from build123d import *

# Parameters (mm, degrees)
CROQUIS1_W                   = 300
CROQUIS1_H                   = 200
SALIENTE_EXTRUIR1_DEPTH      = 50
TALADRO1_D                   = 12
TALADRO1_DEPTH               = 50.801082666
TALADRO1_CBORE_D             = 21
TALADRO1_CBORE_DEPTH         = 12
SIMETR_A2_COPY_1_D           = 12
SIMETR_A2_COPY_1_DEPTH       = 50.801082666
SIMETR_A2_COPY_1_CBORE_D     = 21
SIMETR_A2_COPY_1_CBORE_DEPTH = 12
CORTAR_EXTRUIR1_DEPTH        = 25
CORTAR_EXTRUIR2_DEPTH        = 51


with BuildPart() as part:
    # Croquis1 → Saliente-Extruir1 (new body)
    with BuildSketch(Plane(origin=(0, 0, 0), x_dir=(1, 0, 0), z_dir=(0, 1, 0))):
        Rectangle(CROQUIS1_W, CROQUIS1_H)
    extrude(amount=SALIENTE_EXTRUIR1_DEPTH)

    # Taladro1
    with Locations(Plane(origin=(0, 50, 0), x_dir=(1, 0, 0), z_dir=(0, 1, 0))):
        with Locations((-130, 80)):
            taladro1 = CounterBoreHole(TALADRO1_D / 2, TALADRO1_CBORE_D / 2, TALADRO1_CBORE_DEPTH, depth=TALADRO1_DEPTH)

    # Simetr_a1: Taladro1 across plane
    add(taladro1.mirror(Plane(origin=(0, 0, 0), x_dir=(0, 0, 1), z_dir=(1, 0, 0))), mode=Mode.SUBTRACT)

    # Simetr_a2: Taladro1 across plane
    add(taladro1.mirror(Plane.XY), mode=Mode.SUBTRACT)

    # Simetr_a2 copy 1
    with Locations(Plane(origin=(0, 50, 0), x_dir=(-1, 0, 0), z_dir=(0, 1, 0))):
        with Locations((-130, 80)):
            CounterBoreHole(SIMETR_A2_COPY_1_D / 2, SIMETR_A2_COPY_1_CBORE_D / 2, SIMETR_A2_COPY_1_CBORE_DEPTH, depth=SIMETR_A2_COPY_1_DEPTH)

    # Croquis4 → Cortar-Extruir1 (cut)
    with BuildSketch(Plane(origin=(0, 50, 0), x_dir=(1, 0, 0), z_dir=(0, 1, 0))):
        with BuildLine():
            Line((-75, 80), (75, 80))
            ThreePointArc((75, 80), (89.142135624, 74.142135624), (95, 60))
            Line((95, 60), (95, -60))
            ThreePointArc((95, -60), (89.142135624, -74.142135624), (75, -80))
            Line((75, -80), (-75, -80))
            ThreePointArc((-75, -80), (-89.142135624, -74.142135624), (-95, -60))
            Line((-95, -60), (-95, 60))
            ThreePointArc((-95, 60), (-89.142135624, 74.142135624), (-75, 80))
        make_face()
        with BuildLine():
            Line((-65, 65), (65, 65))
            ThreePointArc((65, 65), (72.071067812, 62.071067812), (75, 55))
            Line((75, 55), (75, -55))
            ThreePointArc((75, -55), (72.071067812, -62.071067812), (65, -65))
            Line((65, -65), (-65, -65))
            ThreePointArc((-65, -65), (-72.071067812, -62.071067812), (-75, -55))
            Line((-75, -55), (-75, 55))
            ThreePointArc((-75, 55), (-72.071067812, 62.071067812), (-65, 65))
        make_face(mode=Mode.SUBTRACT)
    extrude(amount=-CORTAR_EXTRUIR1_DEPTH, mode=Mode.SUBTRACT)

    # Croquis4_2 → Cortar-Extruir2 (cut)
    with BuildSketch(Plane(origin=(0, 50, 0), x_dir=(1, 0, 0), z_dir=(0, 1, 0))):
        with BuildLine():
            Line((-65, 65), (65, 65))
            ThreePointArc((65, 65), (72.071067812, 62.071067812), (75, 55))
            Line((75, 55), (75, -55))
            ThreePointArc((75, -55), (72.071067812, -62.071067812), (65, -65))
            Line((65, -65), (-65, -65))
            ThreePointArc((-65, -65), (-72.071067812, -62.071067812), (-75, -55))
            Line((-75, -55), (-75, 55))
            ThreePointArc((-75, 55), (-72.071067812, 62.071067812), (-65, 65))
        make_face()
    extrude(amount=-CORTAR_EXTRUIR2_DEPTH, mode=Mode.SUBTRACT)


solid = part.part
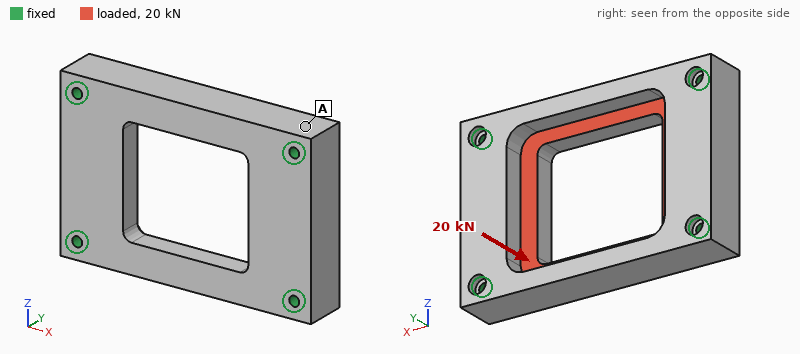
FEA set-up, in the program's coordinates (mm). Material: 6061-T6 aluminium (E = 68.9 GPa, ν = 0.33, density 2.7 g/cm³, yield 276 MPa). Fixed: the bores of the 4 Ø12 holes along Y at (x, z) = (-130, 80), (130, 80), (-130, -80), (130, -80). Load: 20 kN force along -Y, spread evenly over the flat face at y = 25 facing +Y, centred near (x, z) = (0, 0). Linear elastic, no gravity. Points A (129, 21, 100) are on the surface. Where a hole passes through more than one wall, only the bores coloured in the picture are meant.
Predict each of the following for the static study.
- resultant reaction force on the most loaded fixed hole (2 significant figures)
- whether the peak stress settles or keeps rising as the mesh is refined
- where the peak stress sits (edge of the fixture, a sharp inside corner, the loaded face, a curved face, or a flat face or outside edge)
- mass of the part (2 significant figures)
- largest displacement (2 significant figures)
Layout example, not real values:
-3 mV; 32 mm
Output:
5.0 kN; keeps rising; edge of the fixture; 4.7 kg; 43 µm
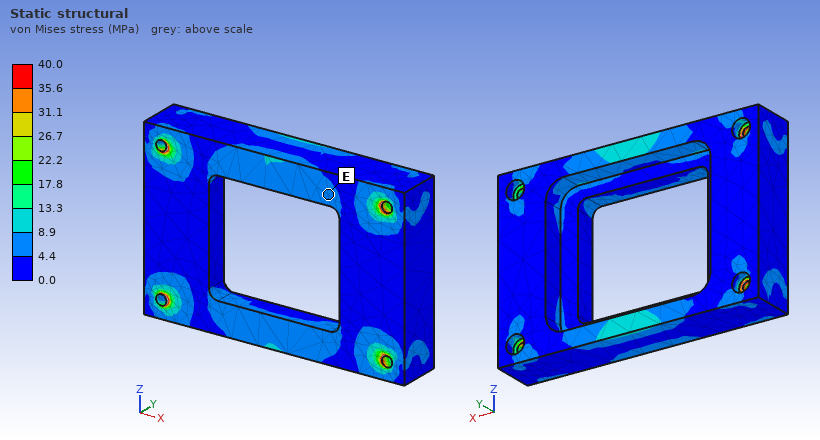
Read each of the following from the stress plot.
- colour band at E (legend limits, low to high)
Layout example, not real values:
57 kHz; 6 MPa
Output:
4.4 to 8.9 MPa
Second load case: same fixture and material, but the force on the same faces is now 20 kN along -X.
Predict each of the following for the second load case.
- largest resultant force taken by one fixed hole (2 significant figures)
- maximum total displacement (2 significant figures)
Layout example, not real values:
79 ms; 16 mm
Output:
5.2 kN; 5.5 µm
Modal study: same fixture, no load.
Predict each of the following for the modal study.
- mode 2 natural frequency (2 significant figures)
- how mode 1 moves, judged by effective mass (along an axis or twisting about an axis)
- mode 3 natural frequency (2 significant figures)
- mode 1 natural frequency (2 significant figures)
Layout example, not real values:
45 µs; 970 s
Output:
3100 Hz; along Y; 3400 Hz; 2900 Hz
